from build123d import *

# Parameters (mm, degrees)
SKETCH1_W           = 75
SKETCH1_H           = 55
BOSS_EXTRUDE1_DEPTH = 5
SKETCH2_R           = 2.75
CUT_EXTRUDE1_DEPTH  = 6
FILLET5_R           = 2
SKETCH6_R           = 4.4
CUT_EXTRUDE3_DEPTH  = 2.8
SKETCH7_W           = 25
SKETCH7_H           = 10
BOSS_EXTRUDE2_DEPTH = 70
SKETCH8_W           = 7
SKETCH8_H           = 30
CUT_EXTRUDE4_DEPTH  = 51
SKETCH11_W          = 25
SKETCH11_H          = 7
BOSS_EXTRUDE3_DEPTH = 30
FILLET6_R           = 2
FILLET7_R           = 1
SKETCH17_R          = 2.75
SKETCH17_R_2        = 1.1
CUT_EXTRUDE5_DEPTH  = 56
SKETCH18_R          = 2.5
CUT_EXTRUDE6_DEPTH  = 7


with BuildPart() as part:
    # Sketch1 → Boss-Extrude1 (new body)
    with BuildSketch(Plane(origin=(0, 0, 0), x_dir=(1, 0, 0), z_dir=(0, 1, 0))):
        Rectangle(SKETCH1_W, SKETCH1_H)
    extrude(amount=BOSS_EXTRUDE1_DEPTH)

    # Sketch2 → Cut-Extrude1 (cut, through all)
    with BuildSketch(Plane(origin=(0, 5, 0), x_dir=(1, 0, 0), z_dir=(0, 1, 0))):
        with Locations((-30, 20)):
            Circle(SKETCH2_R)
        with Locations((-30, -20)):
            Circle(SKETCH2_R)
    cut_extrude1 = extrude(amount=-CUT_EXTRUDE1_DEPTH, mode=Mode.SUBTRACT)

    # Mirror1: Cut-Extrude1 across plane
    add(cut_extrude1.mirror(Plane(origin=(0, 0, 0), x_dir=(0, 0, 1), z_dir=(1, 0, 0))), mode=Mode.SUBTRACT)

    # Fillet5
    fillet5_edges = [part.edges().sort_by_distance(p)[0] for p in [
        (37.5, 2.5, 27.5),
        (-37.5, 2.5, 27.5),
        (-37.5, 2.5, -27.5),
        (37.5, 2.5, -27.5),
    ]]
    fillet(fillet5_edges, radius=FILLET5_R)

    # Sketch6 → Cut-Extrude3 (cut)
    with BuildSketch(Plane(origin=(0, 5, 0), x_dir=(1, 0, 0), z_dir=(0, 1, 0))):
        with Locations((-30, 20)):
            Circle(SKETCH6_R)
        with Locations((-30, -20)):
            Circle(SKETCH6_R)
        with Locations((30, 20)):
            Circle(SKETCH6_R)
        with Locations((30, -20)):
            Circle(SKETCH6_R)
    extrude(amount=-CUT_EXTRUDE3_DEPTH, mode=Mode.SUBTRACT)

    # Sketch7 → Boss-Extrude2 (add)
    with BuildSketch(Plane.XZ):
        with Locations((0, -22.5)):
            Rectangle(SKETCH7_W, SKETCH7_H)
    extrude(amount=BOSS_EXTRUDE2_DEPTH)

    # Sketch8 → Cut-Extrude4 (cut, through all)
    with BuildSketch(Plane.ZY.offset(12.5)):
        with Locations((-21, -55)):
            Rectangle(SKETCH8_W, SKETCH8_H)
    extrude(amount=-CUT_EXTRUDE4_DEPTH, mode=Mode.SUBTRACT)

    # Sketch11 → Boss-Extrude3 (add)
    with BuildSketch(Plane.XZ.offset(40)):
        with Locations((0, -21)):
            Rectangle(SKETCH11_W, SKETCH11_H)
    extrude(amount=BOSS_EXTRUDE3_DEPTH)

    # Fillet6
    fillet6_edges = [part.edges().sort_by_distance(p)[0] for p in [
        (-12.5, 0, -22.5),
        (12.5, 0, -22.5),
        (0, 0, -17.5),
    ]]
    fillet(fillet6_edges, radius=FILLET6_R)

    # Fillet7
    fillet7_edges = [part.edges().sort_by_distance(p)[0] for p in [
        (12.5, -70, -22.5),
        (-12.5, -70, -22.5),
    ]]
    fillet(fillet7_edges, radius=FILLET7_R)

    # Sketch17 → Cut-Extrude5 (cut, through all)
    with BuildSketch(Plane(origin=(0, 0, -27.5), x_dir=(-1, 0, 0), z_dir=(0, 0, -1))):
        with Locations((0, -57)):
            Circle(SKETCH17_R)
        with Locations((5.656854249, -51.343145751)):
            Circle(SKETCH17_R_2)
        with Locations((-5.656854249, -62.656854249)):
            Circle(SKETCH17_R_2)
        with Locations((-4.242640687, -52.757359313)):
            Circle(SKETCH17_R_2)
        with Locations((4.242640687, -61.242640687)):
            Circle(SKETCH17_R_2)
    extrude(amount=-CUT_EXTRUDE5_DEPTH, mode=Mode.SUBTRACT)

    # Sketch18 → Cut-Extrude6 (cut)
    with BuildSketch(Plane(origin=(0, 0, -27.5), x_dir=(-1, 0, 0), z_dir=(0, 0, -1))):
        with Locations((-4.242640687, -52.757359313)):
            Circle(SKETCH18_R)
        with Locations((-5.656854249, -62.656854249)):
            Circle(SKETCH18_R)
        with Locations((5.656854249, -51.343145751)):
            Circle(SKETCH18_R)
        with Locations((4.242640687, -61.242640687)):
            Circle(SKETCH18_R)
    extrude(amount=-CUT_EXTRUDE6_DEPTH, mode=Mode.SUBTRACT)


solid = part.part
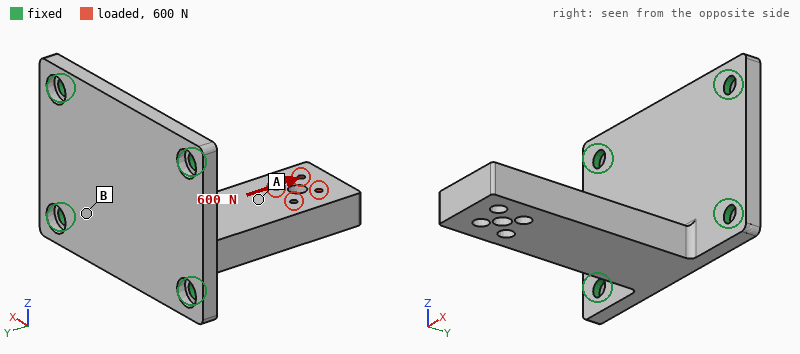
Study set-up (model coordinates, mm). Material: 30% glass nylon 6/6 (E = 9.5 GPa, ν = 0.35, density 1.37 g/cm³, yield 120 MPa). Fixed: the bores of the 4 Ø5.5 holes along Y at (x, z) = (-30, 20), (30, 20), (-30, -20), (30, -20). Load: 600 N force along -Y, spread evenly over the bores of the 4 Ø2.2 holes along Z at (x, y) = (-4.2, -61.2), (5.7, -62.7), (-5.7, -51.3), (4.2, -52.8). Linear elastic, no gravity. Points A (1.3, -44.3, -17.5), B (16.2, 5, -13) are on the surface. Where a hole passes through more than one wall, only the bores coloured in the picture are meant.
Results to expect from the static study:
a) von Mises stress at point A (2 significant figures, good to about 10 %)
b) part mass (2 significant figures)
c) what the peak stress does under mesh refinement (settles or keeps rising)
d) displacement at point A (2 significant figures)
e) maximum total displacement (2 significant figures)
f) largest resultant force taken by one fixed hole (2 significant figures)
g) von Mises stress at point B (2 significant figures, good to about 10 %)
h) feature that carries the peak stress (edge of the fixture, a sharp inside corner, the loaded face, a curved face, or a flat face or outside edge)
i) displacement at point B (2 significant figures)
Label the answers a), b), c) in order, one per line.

a) 7.4 MPa
b) 50 g
c) keeps rising
d) 0.20 mm
e) 0.21 mm
f) 350 N
g) 15 MPa
h) edge of the fixture
i) 0.10 mm
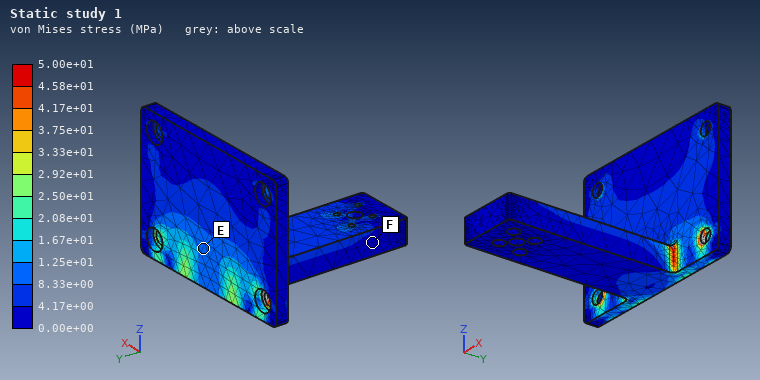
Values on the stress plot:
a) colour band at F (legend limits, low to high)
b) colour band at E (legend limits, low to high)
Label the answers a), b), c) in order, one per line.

a) 0.00e+00 to 4.17e+00 MPa
b) 8.33e+00 to 1.25e+01 MPa
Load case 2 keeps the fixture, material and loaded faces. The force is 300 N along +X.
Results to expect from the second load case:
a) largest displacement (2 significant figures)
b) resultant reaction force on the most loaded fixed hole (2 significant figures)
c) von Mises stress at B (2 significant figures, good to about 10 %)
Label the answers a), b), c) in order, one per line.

a) 0.97 mm
b) 360 N
c) 21 MPa
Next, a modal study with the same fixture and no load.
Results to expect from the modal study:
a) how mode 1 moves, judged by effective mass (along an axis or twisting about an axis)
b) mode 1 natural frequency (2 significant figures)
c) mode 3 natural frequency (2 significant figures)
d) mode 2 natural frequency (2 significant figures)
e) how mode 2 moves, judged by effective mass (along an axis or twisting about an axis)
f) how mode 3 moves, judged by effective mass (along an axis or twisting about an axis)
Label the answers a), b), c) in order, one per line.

a) along Z
b) 470 Hz
c) 1800 Hz
d) 950 Hz
e) along X
f) along Y
